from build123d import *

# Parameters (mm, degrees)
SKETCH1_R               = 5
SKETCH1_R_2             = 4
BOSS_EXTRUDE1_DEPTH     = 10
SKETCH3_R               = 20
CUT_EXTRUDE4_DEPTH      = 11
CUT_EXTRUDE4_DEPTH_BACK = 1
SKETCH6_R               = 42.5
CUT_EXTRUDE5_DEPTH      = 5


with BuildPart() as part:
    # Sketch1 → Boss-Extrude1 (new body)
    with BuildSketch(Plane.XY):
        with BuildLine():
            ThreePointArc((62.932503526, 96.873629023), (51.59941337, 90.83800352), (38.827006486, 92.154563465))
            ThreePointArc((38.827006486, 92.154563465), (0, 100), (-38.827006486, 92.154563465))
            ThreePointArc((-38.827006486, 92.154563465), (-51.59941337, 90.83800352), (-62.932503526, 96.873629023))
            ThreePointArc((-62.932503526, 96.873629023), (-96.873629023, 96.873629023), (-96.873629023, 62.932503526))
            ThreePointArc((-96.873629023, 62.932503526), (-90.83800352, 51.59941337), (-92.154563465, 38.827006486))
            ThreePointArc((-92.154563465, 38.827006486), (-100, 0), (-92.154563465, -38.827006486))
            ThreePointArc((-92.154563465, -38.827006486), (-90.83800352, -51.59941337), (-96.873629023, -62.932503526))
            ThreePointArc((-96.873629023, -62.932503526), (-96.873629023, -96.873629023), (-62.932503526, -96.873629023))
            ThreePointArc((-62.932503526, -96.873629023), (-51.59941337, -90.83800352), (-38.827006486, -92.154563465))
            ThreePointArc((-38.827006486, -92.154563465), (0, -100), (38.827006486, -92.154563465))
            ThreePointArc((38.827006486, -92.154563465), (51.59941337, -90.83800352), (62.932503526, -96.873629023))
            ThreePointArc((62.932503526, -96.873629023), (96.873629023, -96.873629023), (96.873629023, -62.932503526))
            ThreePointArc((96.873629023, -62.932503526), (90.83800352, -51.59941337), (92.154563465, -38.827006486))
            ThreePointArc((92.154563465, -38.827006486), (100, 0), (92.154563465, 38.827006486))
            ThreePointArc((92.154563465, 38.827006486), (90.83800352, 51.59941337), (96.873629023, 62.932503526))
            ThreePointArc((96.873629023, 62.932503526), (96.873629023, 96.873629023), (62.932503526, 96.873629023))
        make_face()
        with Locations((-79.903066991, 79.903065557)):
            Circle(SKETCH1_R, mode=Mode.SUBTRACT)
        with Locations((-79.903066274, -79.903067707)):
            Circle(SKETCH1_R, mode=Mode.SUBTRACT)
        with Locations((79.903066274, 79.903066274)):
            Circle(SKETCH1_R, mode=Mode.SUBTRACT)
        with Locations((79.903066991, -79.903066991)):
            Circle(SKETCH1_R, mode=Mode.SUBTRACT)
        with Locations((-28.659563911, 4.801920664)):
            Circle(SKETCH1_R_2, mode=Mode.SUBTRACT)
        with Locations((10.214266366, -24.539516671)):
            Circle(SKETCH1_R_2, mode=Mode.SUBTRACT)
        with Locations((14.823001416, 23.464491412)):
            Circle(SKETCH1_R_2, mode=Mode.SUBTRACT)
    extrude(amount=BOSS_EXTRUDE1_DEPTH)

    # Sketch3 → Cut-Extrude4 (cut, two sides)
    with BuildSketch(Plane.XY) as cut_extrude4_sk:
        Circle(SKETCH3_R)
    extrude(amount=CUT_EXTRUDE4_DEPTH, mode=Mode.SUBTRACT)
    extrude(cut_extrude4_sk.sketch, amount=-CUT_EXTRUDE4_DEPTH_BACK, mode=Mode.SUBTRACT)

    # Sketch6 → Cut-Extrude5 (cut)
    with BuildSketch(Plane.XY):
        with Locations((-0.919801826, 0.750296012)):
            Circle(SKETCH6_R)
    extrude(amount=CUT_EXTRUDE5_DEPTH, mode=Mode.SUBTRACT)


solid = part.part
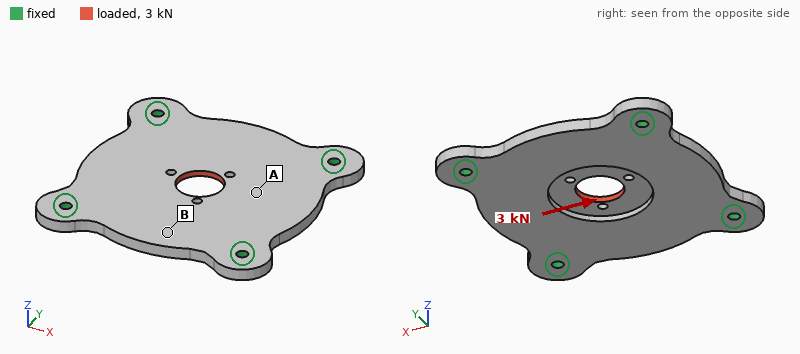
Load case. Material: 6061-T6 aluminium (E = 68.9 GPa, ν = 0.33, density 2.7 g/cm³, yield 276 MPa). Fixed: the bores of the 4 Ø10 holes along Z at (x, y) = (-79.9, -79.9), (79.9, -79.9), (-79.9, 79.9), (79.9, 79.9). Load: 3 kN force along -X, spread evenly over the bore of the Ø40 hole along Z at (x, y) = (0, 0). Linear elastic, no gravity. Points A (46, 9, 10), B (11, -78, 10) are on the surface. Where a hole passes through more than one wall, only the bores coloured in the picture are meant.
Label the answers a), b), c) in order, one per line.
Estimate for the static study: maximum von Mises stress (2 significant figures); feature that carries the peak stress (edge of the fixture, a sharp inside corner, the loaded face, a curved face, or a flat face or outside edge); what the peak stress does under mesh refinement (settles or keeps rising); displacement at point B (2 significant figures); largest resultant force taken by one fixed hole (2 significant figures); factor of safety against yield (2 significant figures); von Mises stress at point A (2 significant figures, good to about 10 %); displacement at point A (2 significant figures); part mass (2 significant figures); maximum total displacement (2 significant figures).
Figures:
a) 17 MPa
b) a curved face
c) settles
d) 1.2 µm
e) 860 N
f) 16
g) 3.1 MPa
h) 3.6 µm
i) 920 g
j) 6.2 µm
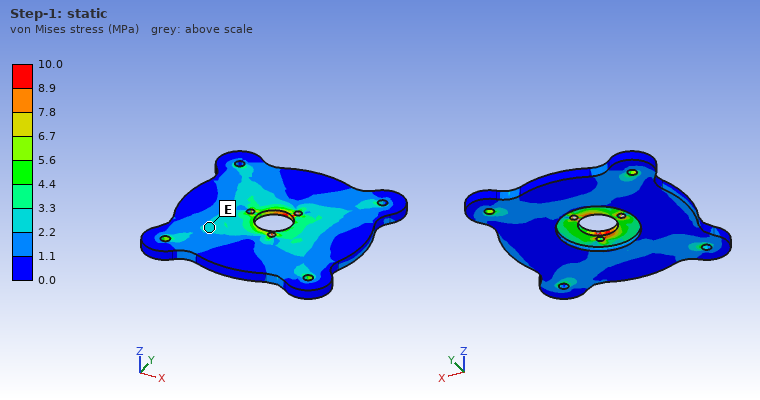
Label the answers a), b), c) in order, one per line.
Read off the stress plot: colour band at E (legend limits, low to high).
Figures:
a) 2.2 to 3.3 MPa
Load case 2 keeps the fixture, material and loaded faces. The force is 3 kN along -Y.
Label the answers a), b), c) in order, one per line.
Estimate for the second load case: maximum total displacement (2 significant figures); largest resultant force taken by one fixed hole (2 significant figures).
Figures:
a) 6.6 µm
b) 870 N
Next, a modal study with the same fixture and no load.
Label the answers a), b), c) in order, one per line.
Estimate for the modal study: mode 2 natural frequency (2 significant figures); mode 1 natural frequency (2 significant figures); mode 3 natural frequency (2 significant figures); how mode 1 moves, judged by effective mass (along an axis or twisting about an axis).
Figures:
a) 2100 Hz
b) 1400 Hz
c) 2100 Hz
d) along Z
